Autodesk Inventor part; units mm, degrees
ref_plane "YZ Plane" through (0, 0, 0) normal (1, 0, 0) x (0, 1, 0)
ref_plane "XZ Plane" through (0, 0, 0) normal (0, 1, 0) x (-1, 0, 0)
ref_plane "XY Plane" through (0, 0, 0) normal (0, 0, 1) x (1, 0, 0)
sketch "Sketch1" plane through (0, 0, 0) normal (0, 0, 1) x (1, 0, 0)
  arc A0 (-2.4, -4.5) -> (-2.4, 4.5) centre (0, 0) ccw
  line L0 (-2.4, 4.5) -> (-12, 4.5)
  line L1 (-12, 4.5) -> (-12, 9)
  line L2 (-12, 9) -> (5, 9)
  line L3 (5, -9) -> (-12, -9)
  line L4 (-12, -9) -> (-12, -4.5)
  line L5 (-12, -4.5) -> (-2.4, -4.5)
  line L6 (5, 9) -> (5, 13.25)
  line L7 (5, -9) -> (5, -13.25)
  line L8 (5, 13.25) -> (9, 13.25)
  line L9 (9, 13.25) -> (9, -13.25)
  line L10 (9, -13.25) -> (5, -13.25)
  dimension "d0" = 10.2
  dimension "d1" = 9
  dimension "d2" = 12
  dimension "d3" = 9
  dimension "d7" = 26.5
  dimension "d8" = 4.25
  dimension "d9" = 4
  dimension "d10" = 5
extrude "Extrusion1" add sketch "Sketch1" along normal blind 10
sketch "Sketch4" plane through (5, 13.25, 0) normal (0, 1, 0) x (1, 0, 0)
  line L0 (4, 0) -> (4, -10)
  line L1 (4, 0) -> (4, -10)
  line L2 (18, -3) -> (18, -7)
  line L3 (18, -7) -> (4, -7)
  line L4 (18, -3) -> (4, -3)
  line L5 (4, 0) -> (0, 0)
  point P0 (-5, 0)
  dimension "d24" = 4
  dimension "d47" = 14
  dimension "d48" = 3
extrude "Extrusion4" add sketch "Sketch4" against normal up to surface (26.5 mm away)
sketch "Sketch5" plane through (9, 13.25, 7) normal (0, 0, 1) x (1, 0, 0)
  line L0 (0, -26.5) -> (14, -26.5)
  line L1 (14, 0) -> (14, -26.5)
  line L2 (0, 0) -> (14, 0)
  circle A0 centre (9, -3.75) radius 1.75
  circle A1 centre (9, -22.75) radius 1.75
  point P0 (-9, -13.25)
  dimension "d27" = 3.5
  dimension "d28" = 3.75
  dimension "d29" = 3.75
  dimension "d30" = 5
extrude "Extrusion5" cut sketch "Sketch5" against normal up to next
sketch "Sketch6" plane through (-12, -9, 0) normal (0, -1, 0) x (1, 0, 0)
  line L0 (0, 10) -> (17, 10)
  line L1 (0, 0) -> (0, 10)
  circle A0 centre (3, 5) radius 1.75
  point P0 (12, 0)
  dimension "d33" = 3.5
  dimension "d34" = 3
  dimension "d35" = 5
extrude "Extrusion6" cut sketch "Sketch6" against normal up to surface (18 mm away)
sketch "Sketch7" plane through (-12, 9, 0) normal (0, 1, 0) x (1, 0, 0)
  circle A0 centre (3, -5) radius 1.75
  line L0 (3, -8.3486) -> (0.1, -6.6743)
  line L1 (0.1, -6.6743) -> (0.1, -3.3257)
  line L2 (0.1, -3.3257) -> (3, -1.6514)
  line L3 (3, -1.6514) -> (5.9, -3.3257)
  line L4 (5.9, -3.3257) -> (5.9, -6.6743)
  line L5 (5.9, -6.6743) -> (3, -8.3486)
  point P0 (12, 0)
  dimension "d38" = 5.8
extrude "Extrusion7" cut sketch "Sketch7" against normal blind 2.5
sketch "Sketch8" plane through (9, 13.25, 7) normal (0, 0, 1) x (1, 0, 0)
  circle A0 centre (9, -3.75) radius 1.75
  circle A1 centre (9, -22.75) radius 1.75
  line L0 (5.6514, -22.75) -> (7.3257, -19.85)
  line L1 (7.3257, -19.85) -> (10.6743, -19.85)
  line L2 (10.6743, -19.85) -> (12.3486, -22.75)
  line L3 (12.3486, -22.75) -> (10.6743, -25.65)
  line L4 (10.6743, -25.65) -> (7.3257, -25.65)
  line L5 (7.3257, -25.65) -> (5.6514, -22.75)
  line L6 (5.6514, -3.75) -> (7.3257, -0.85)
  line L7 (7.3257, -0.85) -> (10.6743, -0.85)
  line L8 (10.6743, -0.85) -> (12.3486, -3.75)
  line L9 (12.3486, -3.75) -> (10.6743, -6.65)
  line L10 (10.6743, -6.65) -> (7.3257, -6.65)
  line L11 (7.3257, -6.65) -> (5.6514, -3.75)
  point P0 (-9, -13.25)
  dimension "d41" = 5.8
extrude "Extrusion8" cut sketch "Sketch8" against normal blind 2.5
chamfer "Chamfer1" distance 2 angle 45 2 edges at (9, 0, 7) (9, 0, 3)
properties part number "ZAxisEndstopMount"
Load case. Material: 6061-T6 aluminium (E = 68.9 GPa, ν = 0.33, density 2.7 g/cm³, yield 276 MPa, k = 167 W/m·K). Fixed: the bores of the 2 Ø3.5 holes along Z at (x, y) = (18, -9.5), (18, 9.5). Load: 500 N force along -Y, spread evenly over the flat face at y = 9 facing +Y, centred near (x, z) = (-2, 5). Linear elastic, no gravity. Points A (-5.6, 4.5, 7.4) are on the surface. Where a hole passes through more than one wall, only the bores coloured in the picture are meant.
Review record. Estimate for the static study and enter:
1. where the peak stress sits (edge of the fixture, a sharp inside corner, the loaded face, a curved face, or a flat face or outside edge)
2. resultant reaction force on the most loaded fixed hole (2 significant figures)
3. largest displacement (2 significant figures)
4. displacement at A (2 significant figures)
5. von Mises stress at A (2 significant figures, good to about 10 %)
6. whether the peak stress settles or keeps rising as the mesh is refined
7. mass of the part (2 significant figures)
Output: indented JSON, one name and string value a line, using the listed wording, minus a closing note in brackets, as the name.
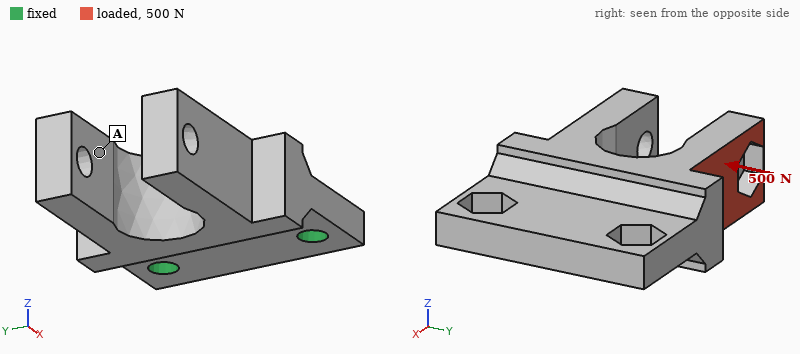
{
  "where the peak stress sits": "edge of the fixture",
  "resultant reaction force on the most loaded fixed hole": "590 N",
  "largest displacement": "79 µm",
  "displacement at A": "45 µm",
  "von Mises stress at A": "15 MPa",
  "whether the peak stress settles or keeps rising as the mesh is refined": "keeps rising",
  "mass of the part": "11 g"
}
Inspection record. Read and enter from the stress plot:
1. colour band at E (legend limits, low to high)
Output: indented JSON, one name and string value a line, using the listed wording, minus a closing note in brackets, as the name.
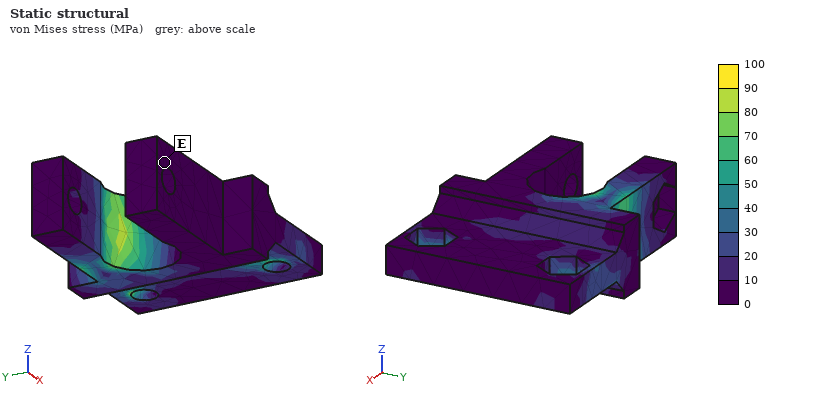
{
  "colour band at E": "0 to 10 MPa"
}
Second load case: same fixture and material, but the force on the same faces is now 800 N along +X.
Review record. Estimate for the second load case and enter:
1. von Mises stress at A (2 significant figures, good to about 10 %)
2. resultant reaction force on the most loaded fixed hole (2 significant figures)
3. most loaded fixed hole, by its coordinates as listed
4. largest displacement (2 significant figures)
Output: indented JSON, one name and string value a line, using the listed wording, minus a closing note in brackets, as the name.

{
  "von Mises stress at A": "11 MPa",
  "resultant reaction force on the most loaded fixed hole": "760 N",
  "most loaded fixed hole, by its coordinates as listed": "(18, 9.5)",
  "largest displacement": "65 µm"
}
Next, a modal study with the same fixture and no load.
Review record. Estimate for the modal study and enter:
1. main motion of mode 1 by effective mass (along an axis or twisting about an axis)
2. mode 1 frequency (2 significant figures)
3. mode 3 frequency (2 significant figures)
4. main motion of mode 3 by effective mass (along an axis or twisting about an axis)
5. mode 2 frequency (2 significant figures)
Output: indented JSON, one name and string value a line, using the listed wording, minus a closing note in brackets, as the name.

{
  "main motion of mode 1 by effective mass": "along Z",
  "mode 1 frequency": "2800 Hz",
  "mode 3 frequency": "11 kHz",
  "main motion of mode 3 by effective mass": "along Y",
  "mode 2 frequency": "9300 Hz"
}
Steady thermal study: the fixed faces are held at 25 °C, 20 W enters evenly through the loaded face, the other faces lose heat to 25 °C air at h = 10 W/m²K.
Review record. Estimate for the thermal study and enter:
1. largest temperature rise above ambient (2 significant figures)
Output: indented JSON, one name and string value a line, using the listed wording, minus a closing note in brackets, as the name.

{
  "largest temperature rise above ambient": "45 K"
}
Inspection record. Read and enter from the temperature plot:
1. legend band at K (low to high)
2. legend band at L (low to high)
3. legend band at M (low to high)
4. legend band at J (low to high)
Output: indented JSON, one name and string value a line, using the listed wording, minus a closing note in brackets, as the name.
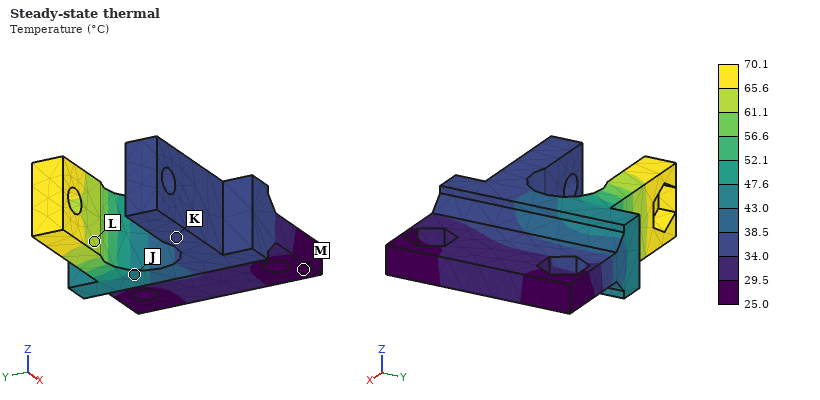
{
  "legend band at K": "34.0 to 38.5 °C",
  "legend band at L": "61.1 to 65.6 °C",
  "legend band at M": "25.0 to 29.5 °C",
  "legend band at J": "43.0 to 47.6 °C"
}
